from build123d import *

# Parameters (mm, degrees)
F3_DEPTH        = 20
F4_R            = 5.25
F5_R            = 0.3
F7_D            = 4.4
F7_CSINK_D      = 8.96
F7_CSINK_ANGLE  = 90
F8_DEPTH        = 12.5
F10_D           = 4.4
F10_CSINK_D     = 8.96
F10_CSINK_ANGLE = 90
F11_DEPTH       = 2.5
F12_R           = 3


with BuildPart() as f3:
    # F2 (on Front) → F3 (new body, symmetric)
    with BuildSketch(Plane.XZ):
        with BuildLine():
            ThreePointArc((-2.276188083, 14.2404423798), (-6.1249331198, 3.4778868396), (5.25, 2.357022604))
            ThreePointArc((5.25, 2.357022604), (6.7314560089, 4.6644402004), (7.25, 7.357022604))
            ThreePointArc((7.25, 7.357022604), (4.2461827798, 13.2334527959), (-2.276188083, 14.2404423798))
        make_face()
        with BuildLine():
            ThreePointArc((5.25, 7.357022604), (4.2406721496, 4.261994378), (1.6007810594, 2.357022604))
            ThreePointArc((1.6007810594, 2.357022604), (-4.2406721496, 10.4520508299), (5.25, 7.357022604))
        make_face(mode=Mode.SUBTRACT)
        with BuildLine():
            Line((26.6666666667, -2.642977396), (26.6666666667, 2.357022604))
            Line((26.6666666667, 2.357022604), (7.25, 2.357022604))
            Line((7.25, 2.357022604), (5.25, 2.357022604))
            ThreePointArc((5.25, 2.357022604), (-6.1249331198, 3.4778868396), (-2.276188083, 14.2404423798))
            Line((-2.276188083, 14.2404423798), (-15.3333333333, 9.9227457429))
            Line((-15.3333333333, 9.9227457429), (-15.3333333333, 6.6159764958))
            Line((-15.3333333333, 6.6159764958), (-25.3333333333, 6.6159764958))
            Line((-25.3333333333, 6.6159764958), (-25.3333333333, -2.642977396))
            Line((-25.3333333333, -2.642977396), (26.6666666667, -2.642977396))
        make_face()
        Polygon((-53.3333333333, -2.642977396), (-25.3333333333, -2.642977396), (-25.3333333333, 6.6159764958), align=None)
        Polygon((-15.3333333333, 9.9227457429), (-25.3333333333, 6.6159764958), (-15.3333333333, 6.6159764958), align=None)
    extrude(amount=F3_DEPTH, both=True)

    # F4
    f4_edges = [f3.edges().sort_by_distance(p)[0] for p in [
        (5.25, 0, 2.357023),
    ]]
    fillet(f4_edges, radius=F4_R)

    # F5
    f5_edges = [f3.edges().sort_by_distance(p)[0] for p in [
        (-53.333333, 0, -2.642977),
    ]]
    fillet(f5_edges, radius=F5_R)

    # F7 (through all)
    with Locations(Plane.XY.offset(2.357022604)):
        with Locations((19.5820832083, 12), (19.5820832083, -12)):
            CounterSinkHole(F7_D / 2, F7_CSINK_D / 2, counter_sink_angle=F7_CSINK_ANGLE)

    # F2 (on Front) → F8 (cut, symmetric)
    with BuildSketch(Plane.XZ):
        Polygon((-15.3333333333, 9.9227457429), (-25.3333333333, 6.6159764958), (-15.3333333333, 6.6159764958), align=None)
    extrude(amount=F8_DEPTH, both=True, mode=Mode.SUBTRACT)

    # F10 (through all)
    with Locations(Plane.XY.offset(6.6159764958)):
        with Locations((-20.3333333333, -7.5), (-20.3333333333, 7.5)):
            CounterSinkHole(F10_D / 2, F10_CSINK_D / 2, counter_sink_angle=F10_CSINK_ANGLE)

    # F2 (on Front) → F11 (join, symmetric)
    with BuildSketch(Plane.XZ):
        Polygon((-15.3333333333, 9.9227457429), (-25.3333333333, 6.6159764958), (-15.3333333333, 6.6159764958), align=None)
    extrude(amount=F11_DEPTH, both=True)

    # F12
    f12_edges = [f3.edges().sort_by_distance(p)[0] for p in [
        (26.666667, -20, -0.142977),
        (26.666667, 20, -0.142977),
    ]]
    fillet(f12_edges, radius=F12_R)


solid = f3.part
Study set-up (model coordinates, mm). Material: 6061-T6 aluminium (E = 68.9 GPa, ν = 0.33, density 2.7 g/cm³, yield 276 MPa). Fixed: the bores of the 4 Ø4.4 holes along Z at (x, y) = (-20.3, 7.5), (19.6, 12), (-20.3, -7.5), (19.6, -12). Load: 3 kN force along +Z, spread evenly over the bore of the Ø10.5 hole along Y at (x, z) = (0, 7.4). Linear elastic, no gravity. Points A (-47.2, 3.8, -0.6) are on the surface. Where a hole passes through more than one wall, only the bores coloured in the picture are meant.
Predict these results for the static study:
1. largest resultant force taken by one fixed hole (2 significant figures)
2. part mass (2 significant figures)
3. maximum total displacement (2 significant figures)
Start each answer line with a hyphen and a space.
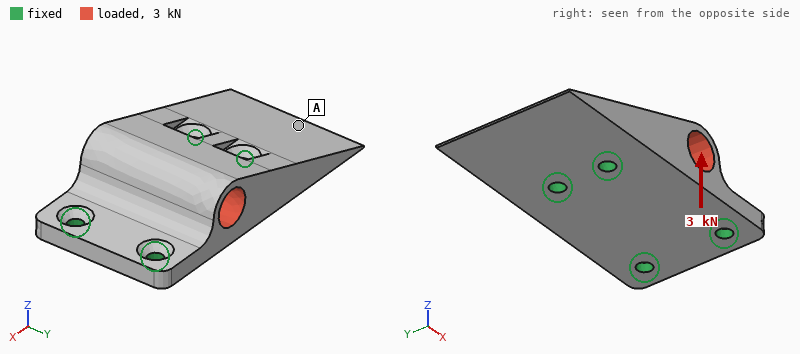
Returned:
- 890 N
- 62 g
- 18 µm
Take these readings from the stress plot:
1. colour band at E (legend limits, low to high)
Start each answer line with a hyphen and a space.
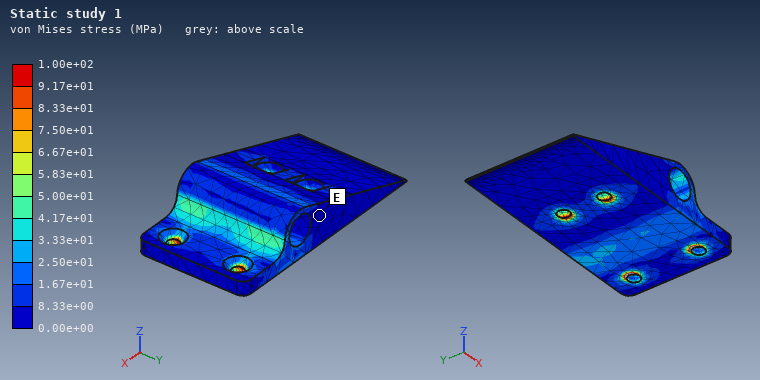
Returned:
- 0.00e+00 to 8.33e+00 MPa
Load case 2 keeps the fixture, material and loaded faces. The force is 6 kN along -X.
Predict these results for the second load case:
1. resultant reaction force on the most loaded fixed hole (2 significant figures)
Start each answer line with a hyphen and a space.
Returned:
- 2.1 kN
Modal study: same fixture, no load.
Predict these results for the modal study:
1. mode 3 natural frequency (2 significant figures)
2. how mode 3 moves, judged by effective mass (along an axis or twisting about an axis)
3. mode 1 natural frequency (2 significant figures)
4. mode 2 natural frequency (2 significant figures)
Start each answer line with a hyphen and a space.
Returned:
- 15 kHz
- along Z
- 10 kHz
- 14 kHz
